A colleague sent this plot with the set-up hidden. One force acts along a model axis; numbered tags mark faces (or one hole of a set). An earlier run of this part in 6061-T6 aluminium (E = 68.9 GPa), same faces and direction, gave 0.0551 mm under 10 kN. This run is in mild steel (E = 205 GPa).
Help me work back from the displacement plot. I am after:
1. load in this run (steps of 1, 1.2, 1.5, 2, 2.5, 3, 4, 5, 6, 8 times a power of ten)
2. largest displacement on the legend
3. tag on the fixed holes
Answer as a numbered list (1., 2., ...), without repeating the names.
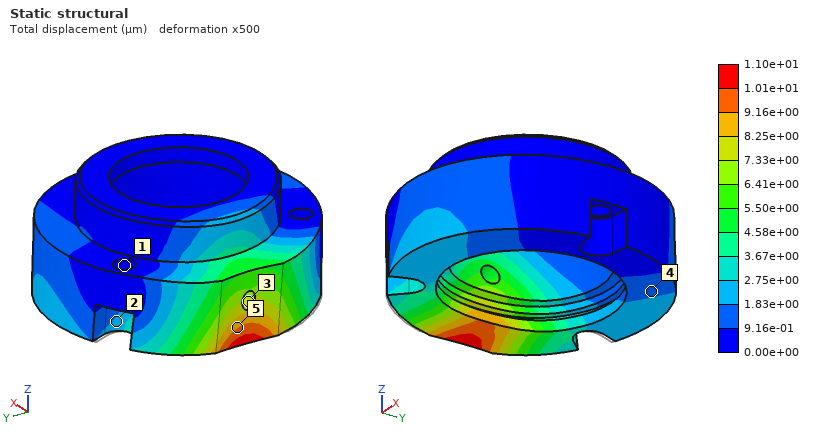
1. 6 kN
2. 1.10e+01 µm
3. 1
